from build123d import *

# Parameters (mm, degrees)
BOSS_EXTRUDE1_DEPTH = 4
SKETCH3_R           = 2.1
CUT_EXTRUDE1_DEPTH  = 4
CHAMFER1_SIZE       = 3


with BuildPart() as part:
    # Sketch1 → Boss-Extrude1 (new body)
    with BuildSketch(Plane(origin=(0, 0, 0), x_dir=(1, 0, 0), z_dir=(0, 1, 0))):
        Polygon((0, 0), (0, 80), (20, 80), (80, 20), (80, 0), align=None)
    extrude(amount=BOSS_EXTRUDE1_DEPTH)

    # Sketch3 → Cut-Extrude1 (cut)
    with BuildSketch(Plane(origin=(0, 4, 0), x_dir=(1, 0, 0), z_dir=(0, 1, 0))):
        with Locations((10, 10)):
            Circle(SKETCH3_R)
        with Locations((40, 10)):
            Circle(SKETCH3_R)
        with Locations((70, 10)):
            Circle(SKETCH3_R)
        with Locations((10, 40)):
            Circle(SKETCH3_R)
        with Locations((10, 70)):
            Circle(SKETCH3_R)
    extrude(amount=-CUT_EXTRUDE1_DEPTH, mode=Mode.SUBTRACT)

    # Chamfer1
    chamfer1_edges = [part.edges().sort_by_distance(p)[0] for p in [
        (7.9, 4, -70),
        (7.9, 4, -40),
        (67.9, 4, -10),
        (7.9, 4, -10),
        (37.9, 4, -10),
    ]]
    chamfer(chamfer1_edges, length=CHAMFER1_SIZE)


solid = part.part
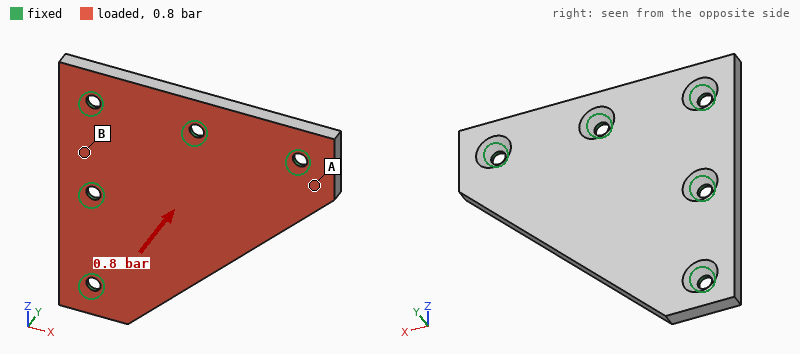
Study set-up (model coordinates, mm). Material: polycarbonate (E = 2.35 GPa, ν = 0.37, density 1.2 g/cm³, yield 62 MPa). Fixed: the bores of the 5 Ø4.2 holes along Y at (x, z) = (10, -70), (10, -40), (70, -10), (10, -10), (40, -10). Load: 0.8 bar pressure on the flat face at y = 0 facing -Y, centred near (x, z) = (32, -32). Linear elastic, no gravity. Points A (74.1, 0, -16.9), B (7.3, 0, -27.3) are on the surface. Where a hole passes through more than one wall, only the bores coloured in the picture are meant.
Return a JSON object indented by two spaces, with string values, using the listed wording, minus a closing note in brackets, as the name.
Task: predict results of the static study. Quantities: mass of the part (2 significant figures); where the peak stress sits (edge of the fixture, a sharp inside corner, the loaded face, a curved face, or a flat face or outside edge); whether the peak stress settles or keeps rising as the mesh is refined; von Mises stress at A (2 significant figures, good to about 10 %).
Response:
{
  "mass of the part": "21 g",
  "where the peak stress sits": "edge of the fixture",
  "whether the peak stress settles or keeps rising as the mesh is refined": "keeps rising",
  "von Mises stress at A": "6.2 MPa"
}
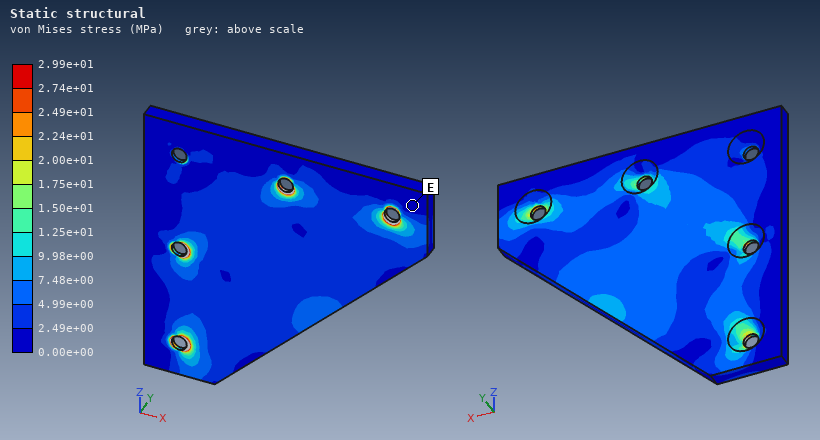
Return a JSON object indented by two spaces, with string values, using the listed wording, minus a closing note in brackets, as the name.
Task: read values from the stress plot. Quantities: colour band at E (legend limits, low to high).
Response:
{
  "colour band at E": "0.00e+00 to 2.49e+00 MPa"
}
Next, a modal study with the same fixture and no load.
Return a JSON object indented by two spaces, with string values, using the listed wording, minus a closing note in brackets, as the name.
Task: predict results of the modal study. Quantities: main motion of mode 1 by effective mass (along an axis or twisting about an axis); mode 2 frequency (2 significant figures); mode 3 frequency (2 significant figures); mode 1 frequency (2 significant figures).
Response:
{
  "main motion of mode 1 by effective mass": "along Y",
  "mode 2 frequency": "1700 Hz",
  "mode 3 frequency": "2800 Hz",
  "mode 1 frequency": "800 Hz"
}
